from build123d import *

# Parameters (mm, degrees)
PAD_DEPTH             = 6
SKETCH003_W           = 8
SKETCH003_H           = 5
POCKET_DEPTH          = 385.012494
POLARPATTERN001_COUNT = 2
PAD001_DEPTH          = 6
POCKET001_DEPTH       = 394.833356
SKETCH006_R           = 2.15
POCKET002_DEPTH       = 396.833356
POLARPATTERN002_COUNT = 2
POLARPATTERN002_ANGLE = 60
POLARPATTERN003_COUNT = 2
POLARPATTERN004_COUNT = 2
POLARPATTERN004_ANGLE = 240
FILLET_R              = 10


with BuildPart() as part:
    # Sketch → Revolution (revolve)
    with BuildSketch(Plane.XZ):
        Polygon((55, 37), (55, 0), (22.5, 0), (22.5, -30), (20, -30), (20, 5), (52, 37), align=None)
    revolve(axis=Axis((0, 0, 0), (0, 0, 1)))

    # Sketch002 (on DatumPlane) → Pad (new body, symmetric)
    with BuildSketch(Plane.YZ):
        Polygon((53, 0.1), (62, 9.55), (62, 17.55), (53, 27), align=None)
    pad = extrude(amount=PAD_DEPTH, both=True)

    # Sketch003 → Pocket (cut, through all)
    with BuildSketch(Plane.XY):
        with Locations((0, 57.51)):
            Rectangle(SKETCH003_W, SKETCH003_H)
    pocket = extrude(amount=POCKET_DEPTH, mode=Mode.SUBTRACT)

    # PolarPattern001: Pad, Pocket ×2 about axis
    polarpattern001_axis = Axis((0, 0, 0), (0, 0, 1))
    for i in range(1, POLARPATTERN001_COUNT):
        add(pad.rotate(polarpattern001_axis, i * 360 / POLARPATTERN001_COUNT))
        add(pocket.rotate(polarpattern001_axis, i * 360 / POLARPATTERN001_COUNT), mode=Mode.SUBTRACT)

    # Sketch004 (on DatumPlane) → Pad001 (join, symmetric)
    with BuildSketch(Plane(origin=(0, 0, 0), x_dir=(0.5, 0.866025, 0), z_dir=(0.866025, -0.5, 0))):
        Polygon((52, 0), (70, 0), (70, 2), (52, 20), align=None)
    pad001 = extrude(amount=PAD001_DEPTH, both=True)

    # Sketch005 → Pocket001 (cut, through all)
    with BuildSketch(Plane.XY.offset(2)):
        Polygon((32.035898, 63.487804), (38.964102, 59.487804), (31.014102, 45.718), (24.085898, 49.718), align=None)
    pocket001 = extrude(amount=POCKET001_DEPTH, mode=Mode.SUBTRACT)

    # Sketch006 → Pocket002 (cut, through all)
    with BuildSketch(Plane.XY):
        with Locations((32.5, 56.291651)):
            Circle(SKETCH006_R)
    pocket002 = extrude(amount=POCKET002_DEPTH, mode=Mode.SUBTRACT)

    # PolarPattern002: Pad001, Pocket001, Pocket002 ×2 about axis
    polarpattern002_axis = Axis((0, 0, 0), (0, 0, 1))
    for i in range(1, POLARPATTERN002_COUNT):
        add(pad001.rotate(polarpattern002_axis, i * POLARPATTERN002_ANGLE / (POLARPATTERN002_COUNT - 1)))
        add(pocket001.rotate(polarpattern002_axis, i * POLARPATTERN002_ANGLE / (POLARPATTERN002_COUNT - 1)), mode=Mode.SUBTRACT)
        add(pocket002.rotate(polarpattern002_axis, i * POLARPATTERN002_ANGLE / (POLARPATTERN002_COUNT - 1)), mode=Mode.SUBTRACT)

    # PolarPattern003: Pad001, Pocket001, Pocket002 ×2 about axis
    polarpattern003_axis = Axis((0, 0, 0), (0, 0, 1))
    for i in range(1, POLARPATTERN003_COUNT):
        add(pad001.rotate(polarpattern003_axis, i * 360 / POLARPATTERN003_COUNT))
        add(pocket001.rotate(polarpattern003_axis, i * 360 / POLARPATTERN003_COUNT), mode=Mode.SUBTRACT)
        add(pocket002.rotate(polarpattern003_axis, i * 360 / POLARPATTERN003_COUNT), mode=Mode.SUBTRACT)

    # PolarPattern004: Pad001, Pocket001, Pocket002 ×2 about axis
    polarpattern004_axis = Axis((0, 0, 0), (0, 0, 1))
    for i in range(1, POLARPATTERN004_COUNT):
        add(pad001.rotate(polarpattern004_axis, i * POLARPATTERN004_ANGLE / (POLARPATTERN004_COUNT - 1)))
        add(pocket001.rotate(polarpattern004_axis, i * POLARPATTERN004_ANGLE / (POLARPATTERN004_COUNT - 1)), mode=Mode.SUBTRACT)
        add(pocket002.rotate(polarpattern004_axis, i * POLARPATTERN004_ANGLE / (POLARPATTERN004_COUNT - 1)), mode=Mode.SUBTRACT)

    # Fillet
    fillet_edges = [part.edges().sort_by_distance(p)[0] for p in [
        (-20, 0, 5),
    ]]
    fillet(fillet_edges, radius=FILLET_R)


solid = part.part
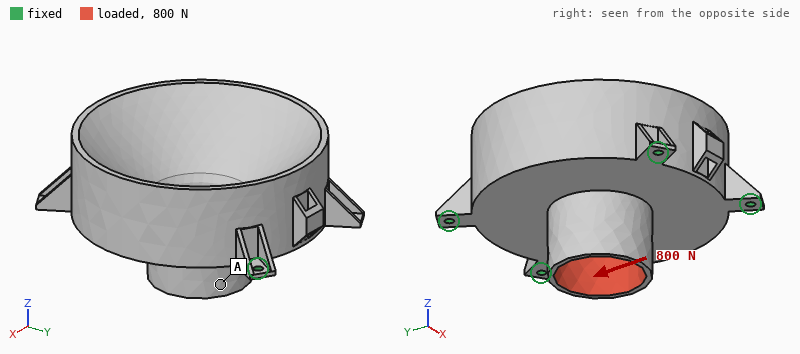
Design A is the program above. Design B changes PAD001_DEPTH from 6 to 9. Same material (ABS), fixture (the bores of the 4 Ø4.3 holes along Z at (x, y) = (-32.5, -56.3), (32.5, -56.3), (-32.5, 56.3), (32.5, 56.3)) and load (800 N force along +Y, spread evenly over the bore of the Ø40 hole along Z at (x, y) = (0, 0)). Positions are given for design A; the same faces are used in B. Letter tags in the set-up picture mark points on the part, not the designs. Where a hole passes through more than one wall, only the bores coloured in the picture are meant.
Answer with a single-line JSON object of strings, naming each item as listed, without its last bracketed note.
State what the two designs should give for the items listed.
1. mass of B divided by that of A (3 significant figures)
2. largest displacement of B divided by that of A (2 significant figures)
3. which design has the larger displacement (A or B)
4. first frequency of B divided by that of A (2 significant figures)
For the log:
{"mass of B divided by that of A": "1.02", "largest displacement of B divided by that of A": "0.89", "which design has the larger displacement": "A", "first frequency of B divided by that of A": "1.2"}
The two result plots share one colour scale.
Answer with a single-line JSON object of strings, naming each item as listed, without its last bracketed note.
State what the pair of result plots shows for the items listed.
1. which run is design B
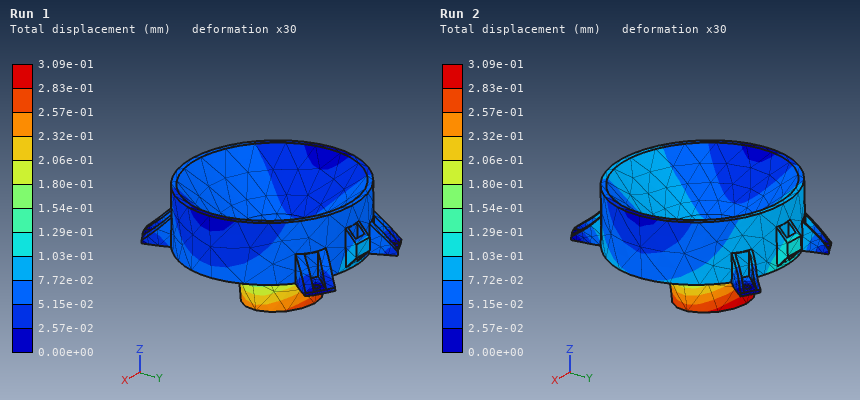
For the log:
{"which run is design B": "Run 1"}
